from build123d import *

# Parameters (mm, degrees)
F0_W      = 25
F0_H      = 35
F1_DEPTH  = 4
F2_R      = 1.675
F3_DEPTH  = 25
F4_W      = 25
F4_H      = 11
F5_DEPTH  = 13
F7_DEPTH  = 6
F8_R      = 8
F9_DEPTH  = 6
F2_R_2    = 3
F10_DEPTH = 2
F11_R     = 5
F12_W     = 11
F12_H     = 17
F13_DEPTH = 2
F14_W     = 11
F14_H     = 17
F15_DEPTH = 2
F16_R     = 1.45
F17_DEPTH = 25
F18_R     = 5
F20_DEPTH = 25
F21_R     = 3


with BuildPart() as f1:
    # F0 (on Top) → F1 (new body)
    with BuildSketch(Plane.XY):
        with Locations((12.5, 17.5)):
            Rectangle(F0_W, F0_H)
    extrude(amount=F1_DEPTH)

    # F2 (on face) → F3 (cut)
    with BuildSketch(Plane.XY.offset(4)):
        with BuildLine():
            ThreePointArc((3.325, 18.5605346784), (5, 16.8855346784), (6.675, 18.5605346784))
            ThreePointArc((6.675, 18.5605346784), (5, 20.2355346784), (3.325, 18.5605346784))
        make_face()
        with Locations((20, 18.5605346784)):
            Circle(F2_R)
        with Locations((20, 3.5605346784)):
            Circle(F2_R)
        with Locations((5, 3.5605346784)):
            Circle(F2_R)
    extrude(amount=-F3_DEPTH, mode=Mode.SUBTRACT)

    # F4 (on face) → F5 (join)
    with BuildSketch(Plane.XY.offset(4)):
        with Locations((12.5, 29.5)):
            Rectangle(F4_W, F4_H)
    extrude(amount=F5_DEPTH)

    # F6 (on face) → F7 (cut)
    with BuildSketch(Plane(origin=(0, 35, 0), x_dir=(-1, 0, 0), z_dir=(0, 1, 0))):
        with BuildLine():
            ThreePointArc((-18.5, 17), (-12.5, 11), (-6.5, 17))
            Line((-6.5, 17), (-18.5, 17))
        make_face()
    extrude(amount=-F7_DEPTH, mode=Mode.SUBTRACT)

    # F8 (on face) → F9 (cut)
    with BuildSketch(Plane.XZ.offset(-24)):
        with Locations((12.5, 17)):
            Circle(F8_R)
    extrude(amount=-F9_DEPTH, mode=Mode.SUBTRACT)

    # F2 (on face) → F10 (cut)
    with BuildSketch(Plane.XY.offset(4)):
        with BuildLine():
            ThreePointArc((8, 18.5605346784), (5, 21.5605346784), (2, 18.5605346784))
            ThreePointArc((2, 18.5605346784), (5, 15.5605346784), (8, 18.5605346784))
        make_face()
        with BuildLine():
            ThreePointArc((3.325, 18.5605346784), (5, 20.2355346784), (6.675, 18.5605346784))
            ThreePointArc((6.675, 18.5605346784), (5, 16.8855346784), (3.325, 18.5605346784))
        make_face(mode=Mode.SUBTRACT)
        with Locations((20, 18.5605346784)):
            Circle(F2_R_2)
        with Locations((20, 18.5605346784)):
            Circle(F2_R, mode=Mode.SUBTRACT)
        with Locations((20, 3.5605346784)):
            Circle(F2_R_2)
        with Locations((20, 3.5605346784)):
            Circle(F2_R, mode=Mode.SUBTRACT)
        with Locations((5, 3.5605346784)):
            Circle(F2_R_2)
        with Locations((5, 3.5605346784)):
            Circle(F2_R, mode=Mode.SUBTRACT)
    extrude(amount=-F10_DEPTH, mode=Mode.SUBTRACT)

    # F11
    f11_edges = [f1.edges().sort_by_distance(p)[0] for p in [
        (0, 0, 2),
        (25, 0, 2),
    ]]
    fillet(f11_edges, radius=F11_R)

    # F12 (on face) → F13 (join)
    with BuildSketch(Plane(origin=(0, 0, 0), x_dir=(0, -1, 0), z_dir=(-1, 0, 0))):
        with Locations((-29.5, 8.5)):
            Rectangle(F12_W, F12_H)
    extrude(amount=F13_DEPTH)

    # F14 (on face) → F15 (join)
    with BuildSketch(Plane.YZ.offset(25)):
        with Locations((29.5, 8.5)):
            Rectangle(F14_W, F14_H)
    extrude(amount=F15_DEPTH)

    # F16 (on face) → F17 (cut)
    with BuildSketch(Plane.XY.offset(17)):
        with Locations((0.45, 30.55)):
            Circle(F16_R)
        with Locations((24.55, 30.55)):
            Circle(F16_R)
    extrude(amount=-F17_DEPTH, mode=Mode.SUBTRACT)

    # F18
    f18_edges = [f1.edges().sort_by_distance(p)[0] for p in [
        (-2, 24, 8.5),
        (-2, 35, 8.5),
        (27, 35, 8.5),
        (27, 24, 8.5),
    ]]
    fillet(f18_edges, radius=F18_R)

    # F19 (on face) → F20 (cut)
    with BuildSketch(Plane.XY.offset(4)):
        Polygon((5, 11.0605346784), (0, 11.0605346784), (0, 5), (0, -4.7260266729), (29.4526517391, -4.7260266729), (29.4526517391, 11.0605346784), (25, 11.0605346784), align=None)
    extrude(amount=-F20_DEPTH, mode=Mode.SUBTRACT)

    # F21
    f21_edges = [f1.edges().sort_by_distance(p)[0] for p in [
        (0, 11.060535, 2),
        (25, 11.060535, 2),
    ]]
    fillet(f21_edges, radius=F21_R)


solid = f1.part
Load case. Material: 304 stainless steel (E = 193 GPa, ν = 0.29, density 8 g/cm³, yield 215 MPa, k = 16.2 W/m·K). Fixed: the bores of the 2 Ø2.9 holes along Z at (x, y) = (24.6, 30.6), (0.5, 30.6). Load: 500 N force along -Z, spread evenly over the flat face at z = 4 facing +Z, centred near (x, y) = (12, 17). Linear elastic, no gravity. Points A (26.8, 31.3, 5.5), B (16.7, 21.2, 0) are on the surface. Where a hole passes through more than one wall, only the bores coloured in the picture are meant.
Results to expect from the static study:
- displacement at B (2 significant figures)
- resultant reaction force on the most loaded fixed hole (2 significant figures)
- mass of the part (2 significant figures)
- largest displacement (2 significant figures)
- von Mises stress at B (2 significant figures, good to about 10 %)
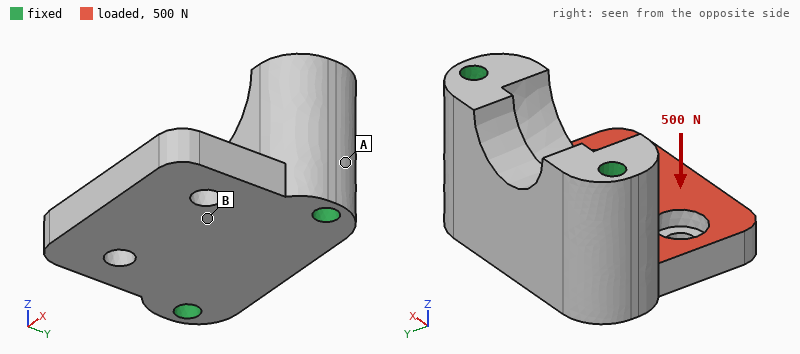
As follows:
3.3 µm
250 N
41 g
13 µm
38 MPa
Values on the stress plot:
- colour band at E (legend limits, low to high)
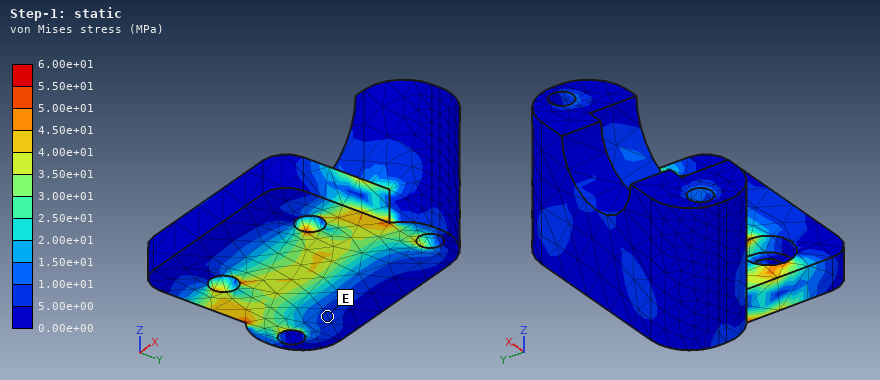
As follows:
5.00e+00 to 1.00e+01 MPa
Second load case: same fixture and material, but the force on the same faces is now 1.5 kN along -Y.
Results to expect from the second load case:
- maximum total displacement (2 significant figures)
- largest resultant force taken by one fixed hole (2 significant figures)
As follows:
12 µm
770 N
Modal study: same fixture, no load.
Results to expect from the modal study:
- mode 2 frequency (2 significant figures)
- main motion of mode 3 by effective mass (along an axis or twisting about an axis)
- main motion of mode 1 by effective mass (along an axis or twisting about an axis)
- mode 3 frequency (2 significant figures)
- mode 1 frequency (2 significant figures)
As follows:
21 kHz
along X
along Z
34 kHz
13 kHz
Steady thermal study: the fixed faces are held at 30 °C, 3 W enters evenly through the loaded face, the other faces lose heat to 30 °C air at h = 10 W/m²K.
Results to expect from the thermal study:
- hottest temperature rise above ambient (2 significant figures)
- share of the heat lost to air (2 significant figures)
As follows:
24 K
5.0 %
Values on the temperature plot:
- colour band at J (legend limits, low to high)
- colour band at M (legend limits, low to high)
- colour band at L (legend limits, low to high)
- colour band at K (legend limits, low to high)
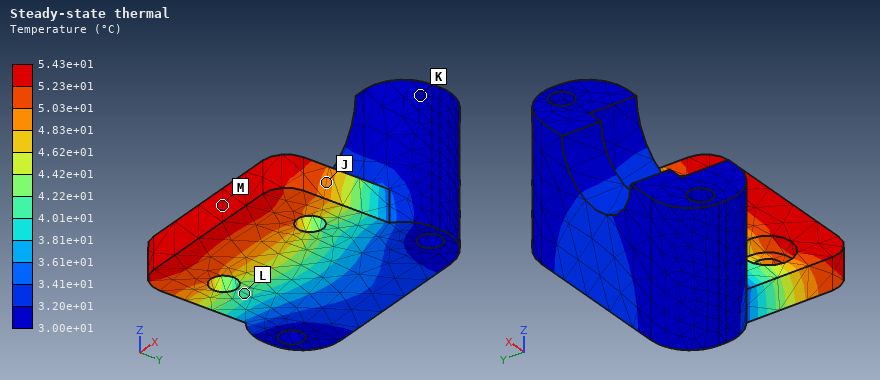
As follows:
4.83e+01 to 5.03e+01 °C
5.23e+01 to 5.43e+01 °C
4.01e+01 to 4.22e+01 °C
3.00e+01 to 3.20e+01 °C
